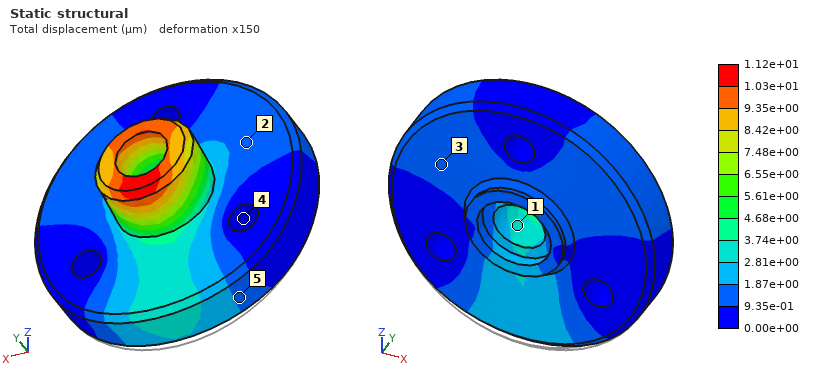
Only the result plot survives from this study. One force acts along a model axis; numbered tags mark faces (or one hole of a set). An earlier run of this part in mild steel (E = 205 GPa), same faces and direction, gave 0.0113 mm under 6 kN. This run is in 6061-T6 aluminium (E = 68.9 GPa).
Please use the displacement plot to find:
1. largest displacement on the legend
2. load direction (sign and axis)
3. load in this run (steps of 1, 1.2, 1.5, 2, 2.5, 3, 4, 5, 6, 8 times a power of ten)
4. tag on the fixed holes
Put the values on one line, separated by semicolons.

1.12e+01 µm; +Z; 2 kN; 4
